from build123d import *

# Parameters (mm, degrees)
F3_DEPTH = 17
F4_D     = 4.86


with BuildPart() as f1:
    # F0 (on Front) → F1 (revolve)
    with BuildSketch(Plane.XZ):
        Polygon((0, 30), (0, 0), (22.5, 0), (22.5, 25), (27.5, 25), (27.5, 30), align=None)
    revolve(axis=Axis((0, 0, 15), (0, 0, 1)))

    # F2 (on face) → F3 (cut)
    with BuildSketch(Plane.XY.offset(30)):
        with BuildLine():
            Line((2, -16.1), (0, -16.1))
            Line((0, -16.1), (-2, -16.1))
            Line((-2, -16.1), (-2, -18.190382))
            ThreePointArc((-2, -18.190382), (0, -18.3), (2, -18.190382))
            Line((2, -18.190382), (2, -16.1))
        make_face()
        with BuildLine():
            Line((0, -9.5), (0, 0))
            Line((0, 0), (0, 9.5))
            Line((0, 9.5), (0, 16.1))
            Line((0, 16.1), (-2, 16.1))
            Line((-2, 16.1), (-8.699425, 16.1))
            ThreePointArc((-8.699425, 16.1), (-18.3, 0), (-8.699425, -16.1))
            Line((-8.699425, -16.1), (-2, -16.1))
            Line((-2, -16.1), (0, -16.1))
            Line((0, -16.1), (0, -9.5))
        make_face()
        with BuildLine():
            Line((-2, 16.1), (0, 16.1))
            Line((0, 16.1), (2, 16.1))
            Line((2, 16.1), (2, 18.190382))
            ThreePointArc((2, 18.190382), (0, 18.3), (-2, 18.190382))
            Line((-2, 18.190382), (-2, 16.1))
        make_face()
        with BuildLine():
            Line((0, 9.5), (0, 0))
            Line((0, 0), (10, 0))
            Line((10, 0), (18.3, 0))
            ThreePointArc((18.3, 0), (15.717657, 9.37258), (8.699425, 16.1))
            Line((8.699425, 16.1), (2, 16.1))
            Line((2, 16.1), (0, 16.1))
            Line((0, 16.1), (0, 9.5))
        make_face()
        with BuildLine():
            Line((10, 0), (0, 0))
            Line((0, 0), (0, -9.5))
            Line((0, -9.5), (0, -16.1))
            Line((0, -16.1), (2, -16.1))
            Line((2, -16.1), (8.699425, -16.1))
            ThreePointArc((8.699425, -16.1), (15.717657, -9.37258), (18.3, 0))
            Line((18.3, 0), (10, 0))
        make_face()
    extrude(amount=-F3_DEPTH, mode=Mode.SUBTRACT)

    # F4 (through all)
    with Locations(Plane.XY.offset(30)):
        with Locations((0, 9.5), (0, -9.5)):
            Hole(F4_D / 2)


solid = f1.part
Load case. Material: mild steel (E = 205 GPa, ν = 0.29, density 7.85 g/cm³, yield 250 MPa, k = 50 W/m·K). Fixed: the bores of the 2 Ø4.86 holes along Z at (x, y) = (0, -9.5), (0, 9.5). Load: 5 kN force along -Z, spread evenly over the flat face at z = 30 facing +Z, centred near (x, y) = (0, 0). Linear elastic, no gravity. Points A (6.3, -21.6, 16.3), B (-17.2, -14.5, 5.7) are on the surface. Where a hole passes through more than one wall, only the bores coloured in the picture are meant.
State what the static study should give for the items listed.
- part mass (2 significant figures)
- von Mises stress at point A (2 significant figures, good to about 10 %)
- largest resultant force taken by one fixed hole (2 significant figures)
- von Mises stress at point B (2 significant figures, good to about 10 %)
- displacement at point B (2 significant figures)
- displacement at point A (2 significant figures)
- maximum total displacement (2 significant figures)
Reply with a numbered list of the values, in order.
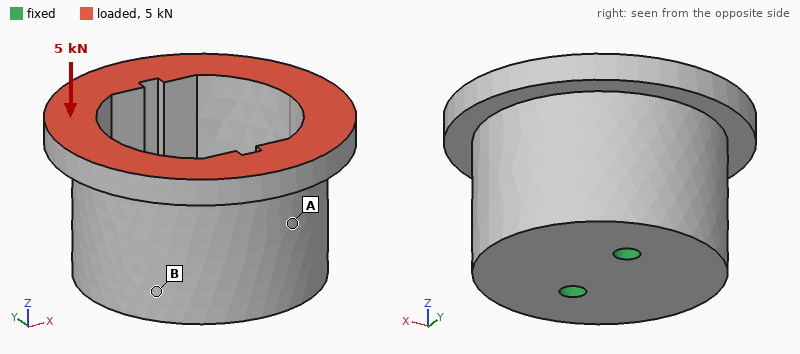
1. 270 g
2. 7.7 MPa
3. 2.5 kN
4. 3.2 MPa
5. 1.8 µm
6. 1.4 µm
7. 5.0 µm
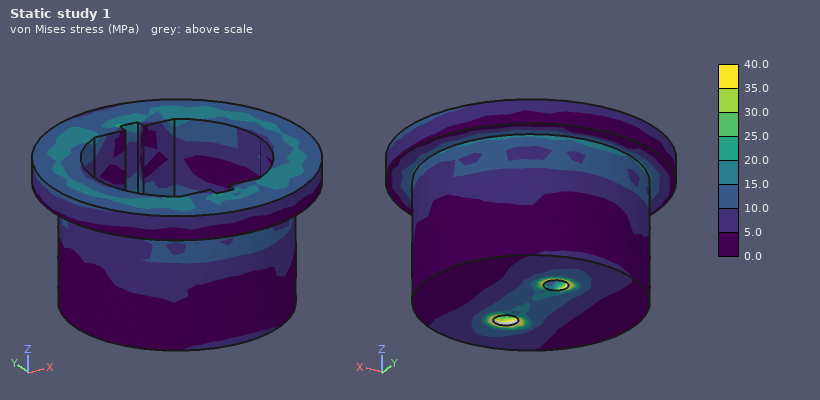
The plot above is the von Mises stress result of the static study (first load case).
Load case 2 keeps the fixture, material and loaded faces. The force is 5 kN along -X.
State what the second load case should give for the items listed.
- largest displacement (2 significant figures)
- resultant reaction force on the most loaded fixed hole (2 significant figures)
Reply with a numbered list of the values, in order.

1. 24 µm
2. 2.5 kN
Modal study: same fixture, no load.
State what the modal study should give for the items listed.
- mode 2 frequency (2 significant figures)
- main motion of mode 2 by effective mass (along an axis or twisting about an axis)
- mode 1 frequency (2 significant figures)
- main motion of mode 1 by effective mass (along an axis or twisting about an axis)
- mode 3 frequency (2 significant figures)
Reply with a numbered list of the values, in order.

1. 12 kHz
2. along Y
3. 8900 Hz
4. along X
5. 13 kHz
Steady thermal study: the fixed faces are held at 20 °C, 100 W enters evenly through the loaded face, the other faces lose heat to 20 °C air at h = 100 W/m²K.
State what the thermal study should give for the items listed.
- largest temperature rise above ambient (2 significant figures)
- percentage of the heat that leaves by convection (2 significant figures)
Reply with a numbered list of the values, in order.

1. 71 K
2. 33 %
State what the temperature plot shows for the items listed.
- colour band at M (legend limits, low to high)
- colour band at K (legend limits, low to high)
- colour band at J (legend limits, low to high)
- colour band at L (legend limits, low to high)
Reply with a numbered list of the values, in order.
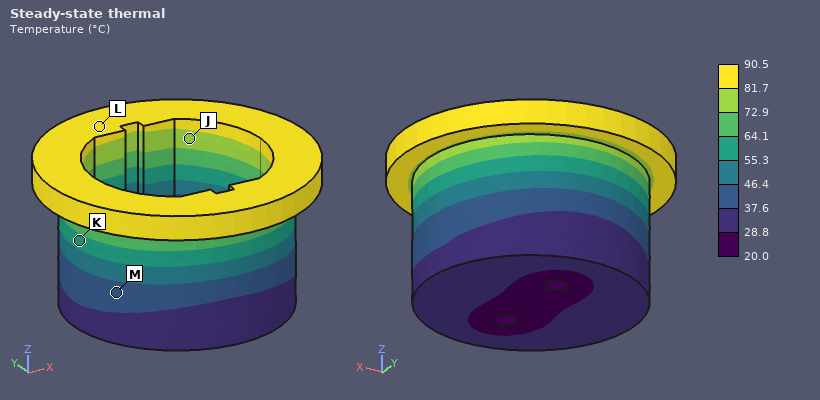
1. 37.6 to 46.4 °C
2. 55.3 to 64.1 °C
3. 72.9 to 81.7 °C
4. 81.7 to 90.5 °C
